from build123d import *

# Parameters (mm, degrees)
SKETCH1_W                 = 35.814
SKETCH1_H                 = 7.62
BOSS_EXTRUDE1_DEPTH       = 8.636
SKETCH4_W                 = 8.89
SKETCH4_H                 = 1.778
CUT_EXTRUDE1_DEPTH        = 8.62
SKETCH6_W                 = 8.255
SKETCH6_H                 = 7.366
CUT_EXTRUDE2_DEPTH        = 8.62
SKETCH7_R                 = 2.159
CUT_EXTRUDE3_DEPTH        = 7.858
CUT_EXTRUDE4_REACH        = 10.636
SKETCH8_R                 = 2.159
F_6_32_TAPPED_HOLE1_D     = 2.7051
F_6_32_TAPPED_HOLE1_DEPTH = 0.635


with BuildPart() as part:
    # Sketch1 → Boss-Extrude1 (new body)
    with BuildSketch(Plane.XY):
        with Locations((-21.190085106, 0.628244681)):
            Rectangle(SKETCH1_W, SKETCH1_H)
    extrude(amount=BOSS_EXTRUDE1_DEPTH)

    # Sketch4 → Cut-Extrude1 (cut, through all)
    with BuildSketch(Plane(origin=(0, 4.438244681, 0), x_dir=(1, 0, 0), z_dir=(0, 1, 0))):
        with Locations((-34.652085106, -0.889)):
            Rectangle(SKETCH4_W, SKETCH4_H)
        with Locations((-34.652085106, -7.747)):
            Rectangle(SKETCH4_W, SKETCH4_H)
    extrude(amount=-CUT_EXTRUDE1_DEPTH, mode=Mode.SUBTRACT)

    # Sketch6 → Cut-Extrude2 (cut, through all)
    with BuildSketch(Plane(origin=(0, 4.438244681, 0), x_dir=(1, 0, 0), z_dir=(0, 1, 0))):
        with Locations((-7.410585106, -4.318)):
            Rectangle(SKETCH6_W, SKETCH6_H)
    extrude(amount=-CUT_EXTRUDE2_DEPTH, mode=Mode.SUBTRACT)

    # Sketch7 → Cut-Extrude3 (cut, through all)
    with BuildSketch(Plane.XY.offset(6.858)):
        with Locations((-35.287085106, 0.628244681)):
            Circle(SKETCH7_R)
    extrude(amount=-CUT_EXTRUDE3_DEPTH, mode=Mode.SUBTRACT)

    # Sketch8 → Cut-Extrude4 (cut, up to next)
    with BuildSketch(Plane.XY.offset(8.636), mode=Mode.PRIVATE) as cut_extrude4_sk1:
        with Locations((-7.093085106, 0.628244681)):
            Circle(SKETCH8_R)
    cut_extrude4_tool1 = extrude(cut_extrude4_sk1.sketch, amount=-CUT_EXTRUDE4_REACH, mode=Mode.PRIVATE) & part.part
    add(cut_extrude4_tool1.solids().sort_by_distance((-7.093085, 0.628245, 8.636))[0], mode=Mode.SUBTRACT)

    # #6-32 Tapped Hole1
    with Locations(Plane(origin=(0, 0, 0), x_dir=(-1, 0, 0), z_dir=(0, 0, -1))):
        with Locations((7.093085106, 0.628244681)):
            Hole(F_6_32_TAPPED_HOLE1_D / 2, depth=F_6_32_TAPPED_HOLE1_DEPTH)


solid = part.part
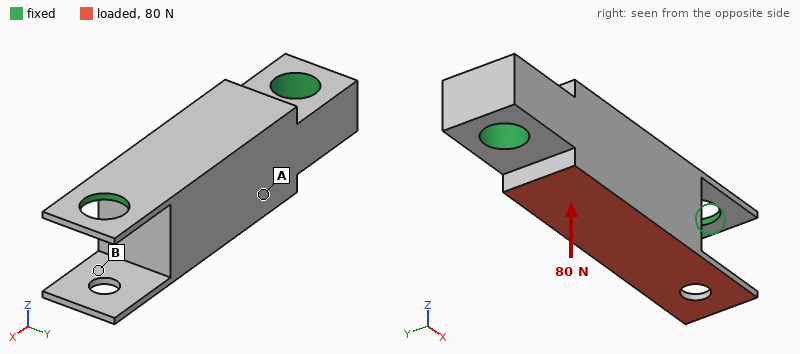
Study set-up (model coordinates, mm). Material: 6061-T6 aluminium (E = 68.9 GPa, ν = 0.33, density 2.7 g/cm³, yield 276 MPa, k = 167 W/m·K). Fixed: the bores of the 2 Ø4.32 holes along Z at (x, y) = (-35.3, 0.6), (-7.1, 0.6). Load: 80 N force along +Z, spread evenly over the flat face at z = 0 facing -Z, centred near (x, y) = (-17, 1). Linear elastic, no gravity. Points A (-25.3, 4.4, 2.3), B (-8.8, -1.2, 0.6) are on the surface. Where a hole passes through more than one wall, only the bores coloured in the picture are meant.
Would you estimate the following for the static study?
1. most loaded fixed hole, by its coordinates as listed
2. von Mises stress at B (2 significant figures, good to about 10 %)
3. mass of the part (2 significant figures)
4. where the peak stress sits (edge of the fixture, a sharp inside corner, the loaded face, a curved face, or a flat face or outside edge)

(-35.3, 0.6)
91 MPa
4.2 g
the loaded face
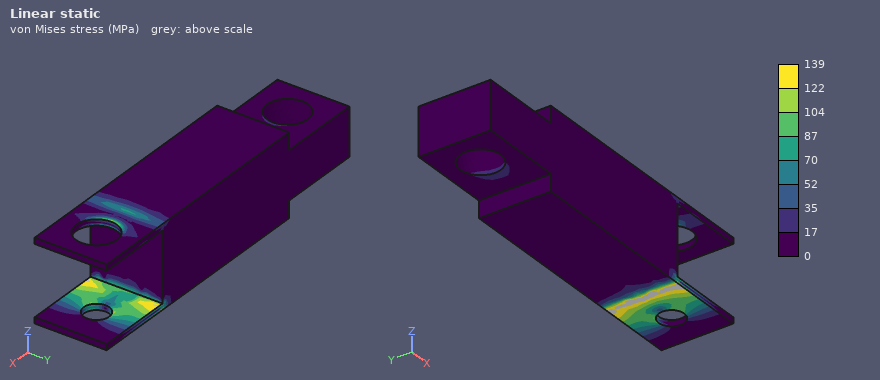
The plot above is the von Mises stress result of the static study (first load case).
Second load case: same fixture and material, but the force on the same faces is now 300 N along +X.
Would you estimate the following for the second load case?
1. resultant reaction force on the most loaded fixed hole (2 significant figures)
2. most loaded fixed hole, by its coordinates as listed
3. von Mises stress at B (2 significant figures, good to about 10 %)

330 N
(-35.3, 0.6)
21 MPa
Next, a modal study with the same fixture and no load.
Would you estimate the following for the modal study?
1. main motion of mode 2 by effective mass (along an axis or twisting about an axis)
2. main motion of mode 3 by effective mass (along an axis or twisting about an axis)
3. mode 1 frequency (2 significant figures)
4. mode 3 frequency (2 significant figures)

along Z
along Y
7000 Hz
16 kHz
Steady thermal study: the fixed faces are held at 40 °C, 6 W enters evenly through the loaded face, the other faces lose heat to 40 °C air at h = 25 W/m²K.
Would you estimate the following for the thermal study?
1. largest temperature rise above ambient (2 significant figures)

20 K
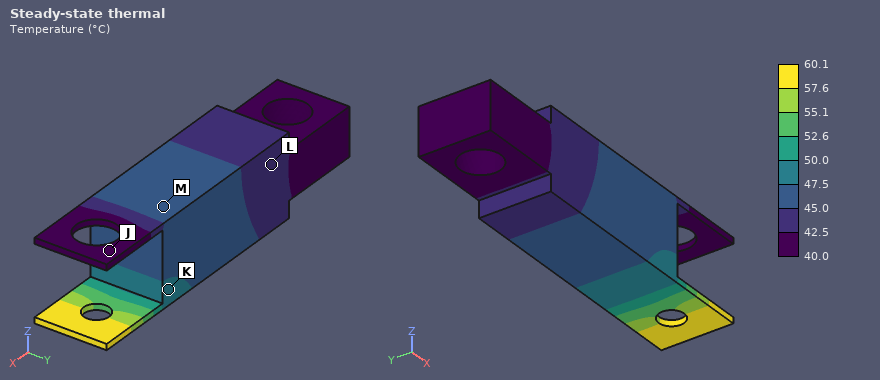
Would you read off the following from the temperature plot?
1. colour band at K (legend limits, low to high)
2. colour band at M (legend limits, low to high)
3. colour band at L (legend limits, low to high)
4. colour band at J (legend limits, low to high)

47.5 to 50.0 °C
45.0 to 47.5 °C
42.5 to 45.0 °C
40.0 to 42.5 °C
